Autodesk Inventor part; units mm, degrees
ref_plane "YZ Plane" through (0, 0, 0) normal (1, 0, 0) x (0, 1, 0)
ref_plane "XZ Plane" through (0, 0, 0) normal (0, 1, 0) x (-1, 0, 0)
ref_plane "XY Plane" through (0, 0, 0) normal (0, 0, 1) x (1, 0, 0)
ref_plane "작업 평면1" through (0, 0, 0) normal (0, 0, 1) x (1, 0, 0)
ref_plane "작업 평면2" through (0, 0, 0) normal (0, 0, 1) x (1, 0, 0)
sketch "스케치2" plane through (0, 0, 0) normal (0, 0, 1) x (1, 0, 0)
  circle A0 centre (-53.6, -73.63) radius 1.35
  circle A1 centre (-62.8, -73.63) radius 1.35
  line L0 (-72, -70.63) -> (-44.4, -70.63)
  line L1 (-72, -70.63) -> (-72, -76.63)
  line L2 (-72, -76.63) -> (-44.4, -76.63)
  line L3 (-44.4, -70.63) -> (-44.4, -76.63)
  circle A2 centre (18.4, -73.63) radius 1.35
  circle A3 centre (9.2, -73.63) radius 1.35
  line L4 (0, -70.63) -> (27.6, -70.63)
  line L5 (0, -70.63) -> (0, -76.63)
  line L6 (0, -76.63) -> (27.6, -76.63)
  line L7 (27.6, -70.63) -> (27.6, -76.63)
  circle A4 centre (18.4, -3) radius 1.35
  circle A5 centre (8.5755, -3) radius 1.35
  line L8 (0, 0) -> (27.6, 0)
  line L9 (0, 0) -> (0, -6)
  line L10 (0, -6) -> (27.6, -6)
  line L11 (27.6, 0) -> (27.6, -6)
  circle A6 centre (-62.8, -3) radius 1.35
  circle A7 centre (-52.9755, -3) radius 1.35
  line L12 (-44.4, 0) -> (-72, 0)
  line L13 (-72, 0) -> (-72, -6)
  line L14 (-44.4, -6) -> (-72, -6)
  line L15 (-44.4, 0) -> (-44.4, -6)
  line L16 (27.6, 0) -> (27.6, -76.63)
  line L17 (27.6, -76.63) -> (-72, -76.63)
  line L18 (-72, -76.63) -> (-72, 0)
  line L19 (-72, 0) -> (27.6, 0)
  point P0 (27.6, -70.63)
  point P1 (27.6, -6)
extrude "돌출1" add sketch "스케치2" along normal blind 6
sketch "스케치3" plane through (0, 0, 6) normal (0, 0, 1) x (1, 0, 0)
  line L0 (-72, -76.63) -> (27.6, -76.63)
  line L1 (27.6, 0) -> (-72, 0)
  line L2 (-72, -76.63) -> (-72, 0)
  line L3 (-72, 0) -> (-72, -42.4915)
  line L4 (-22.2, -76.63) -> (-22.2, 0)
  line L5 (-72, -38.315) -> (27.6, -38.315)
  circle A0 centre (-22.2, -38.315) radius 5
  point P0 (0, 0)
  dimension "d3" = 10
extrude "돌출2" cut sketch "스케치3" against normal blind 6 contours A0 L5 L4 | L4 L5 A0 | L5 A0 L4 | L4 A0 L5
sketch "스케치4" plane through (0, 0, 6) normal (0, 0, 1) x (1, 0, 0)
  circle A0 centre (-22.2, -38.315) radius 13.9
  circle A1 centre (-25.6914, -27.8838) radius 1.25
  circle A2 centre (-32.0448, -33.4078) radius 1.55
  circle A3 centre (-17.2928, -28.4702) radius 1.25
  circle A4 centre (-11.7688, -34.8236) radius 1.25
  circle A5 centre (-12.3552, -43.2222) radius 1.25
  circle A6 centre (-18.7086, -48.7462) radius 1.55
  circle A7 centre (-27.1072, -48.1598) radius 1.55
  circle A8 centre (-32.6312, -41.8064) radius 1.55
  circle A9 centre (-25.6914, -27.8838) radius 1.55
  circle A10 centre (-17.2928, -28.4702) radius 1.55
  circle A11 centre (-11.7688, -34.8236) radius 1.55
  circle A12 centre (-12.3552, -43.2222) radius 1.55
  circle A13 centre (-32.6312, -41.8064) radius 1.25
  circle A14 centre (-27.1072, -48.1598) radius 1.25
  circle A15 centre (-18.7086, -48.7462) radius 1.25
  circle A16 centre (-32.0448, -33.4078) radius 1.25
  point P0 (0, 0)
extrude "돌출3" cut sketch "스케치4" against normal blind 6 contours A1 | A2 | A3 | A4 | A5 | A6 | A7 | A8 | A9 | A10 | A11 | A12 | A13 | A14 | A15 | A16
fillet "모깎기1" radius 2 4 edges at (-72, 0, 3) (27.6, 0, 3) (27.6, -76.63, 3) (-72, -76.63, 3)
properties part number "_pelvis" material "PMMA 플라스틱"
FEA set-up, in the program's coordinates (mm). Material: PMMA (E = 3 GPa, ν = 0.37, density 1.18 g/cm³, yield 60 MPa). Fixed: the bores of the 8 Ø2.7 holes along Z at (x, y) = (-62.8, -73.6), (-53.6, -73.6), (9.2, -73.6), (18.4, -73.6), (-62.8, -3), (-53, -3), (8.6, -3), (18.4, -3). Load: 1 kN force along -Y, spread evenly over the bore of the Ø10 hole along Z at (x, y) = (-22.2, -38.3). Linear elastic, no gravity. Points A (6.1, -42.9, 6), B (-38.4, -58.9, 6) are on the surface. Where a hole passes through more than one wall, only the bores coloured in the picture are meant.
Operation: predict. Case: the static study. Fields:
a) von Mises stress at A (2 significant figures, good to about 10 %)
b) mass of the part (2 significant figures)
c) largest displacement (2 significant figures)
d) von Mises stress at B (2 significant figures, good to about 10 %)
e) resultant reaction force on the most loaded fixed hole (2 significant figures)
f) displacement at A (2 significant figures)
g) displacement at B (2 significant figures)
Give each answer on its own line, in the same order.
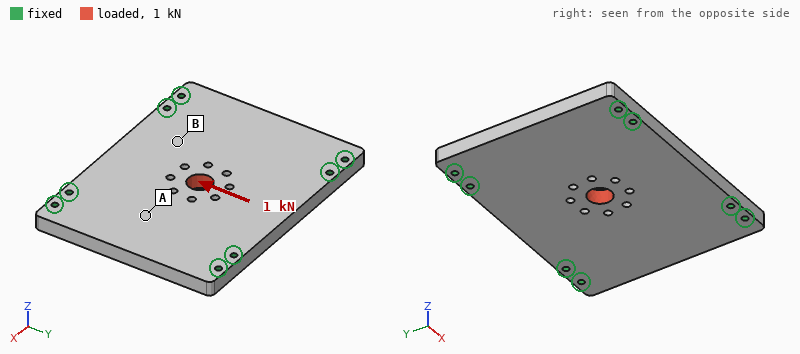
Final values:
1.1 MPa
53 g
57 µm
2.4 MPa
200 N
15 µm
25 µm
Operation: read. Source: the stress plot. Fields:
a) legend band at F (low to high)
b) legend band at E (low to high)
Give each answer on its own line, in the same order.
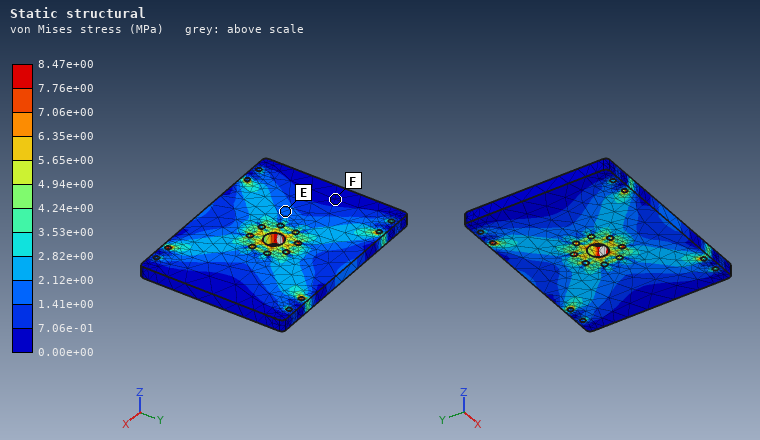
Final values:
0.00e+00 to 7.06e-01 MPa
1.41e+00 to 2.12e+00 MPa
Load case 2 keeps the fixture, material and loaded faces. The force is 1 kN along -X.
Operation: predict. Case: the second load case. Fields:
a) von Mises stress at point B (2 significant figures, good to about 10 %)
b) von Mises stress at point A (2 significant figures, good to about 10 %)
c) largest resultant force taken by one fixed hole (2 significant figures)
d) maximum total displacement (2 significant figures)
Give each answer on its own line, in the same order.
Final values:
2.0 MPa
1.0 MPa
180 N
55 µm
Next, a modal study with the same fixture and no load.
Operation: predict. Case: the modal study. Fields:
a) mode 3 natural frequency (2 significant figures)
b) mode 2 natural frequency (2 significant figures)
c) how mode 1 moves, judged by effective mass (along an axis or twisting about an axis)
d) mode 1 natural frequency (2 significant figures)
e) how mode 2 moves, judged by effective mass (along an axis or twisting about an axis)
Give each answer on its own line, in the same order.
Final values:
2100 Hz
1900 Hz
along Z
1300 Hz
twisting about Y
